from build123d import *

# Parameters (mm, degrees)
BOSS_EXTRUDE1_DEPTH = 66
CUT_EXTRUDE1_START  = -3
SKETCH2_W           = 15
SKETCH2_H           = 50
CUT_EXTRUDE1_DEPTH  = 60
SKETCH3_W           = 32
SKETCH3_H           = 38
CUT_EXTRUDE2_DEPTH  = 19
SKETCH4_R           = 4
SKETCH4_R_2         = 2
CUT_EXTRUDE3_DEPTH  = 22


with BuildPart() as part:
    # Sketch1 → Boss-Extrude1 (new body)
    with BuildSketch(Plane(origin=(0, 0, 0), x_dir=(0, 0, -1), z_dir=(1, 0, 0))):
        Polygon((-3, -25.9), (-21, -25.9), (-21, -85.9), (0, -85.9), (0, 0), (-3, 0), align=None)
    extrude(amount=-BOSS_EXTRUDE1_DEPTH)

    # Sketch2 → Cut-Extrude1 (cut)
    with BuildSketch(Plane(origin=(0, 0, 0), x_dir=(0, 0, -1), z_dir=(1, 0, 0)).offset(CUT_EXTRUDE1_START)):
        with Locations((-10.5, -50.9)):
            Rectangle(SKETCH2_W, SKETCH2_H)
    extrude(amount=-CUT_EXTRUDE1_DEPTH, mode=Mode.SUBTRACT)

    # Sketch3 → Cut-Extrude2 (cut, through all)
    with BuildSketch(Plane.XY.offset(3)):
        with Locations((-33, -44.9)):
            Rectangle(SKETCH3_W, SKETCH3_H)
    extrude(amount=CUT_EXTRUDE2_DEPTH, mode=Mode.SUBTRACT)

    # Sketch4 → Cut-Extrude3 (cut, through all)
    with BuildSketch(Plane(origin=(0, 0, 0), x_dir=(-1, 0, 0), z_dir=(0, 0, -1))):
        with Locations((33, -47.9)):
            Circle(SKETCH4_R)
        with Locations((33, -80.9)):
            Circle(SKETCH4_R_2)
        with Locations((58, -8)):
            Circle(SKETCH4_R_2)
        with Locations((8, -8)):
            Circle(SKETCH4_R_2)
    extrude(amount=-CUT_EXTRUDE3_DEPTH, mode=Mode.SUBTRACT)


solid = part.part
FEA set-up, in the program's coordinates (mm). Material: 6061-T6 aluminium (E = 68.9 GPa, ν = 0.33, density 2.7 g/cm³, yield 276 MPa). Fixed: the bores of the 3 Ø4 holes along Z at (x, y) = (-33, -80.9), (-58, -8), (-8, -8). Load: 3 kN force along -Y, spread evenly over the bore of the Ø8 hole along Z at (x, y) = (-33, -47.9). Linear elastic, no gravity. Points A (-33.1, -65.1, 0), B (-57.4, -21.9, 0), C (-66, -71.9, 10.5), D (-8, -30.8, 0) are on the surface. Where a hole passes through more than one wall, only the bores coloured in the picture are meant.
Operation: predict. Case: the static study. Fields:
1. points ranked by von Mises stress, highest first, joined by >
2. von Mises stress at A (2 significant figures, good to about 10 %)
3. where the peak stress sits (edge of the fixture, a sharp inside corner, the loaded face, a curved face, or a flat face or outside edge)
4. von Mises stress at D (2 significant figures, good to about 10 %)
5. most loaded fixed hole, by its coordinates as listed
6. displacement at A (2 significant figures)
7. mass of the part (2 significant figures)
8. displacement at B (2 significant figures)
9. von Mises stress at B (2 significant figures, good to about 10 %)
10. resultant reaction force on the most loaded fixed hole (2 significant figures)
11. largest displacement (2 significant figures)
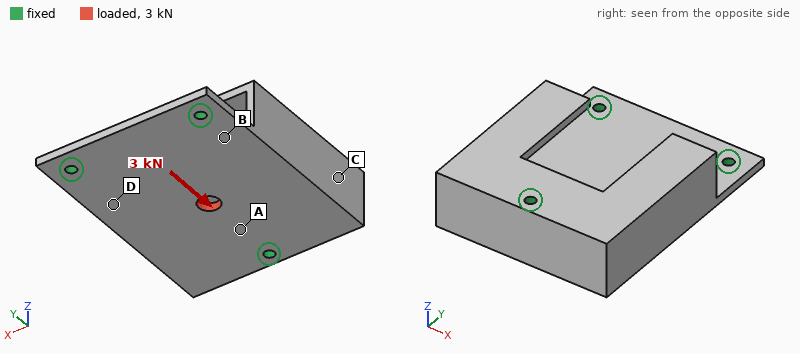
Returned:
A > B > D > C
24 MPa
the loaded face
7.3 MPa
(-33, -80.9)
6.3 µm
110 g
3.3 µm
13 MPa
1.5 kN
13 µm
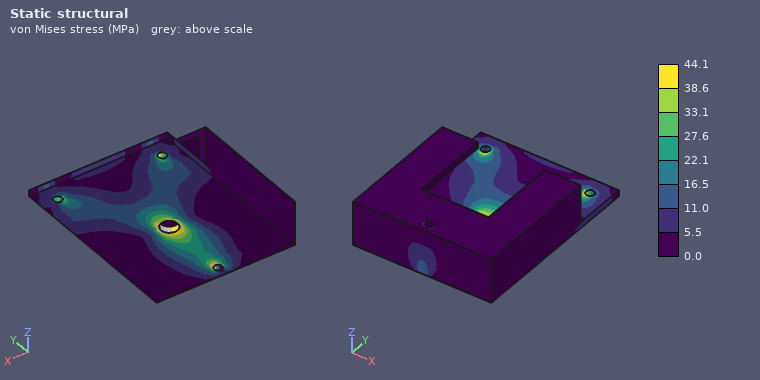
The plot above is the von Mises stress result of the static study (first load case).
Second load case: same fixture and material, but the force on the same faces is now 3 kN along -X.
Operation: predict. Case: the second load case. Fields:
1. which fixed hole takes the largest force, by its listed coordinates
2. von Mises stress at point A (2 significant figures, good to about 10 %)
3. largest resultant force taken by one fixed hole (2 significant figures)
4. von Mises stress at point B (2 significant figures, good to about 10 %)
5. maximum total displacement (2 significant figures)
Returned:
(-33, -80.9)
12 MPa
1.4 kN
14 MPa
18 µm
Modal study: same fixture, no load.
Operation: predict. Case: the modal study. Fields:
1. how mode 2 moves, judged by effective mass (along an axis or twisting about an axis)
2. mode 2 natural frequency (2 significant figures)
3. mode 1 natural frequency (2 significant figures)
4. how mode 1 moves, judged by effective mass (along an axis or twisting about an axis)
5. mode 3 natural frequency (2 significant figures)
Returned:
twisting about Y
3800 Hz
3400 Hz
along Z
5200 Hz
